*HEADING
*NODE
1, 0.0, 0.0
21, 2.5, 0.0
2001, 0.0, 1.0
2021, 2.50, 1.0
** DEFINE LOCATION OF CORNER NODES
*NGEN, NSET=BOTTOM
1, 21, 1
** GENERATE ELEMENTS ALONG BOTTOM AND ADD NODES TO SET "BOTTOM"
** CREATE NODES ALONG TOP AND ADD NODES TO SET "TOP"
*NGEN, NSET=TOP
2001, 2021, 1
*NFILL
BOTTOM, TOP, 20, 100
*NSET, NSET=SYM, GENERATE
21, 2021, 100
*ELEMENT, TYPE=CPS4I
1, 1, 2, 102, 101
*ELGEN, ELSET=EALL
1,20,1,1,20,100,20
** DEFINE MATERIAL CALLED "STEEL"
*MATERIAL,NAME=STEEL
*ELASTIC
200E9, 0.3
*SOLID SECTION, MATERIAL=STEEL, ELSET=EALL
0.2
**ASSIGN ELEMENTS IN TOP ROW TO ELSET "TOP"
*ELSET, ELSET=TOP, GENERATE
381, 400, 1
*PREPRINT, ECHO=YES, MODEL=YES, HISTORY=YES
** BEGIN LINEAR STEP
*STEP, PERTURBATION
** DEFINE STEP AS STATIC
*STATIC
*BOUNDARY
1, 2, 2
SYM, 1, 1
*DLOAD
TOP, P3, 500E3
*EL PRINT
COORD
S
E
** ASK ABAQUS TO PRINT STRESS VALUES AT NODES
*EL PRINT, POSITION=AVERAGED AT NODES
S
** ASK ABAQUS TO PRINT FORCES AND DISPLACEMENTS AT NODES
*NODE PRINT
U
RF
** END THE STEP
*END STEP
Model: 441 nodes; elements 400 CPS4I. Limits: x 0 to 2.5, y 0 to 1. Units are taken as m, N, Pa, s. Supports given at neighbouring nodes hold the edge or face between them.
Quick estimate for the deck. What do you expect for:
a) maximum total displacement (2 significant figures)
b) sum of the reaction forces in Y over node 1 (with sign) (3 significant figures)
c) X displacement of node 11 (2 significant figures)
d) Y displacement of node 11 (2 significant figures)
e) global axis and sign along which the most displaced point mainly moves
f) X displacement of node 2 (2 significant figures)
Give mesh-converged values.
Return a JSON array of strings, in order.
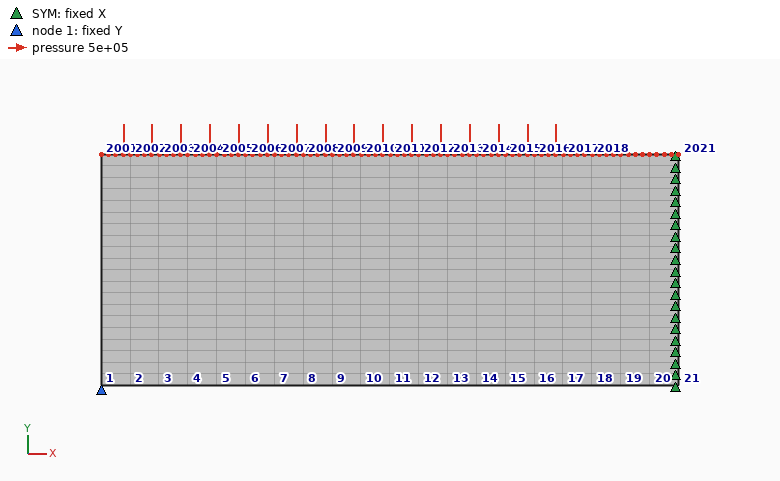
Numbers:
["3.3e-04 m", "2.50e+05 N", "-5.4e-05 m", "-2.5e-04 m", "-Y", "-8.9e-05 m"]
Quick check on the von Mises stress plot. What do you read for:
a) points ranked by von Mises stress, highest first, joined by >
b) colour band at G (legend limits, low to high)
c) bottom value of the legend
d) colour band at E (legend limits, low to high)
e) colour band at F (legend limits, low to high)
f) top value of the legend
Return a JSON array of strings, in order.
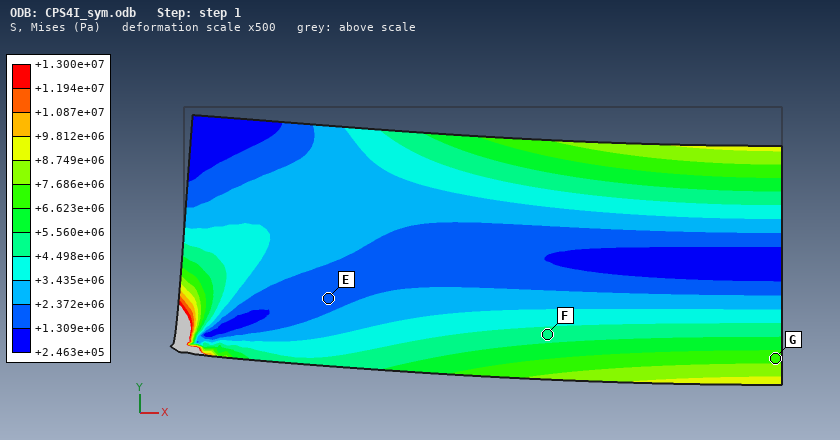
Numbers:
["G > F > E", "+6.623e+06 to +7.686e+06 Pa", "+2.463e+05 Pa", "+1.309e+06 to +2.372e+06 Pa", "+4.498e+06 to +5.560e+06 Pa", "+1.300e+07 Pa"]
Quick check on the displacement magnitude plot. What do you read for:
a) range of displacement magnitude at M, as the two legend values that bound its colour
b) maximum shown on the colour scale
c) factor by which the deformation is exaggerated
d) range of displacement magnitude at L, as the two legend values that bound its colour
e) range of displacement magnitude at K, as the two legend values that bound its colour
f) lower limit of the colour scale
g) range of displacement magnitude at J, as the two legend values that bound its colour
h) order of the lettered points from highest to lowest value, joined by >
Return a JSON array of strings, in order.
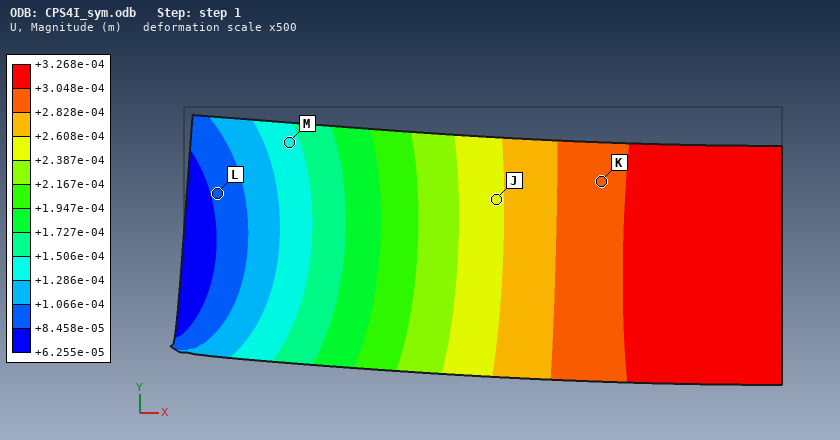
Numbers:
["+1.286e-04 to +1.506e-04 m", "+3.268e-04 m", "500", "+8.458e-05 to +1.066e-04 m", "+2.828e-04 to +3.048e-04 m", "+6.255e-05 m", "+2.387e-04 to +2.608e-04 m", "K > J > M > L"]
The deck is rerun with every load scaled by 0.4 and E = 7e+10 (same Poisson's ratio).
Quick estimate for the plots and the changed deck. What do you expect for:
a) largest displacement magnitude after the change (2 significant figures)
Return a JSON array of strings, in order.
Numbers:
["3.7e-04 m"]
